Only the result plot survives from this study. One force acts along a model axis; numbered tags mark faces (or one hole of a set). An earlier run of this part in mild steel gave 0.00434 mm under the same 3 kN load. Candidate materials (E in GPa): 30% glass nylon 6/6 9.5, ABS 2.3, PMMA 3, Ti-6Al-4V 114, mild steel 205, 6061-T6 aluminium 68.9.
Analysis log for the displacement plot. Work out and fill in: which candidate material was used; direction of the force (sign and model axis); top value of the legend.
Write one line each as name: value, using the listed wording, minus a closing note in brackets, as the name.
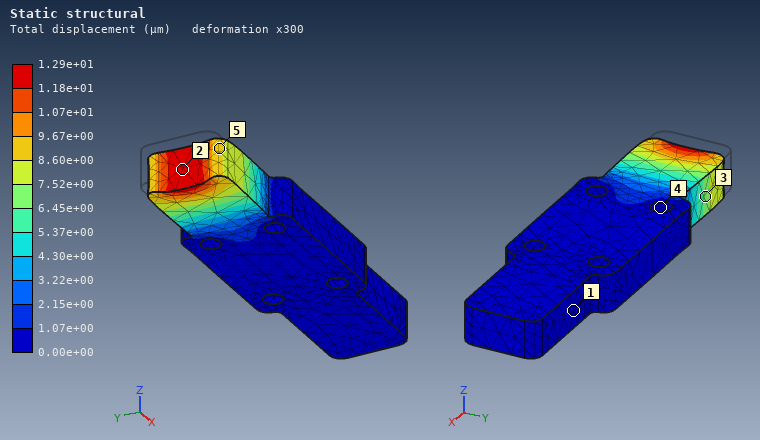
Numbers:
which candidate material was used: 6061-T6 aluminium
direction of the force: +X
top value of the legend: 1.29e+01 µm
